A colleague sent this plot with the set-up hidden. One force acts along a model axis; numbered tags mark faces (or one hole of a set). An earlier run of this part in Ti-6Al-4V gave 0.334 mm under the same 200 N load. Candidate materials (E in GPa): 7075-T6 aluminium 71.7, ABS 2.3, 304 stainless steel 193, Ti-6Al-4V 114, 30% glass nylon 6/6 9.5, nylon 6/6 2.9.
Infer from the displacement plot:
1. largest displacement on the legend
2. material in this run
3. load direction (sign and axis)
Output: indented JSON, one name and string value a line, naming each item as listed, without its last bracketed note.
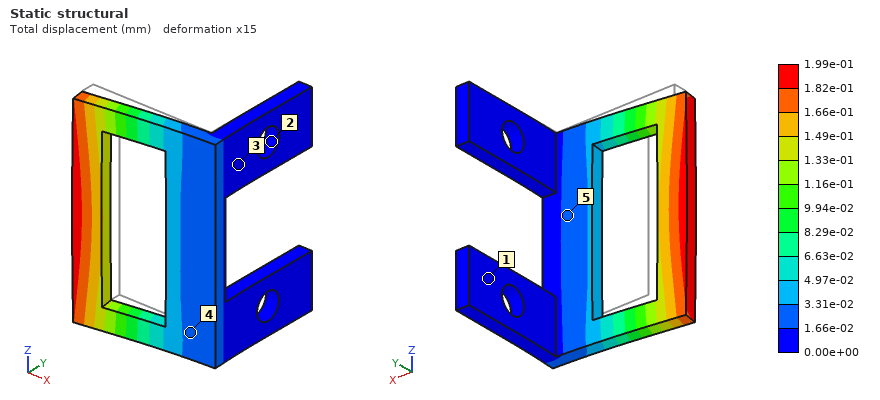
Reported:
{
  "largest displacement on the legend": "1.99e-01 mm",
  "material in this run": "304 stainless steel",
  "load direction": "-Y"
}
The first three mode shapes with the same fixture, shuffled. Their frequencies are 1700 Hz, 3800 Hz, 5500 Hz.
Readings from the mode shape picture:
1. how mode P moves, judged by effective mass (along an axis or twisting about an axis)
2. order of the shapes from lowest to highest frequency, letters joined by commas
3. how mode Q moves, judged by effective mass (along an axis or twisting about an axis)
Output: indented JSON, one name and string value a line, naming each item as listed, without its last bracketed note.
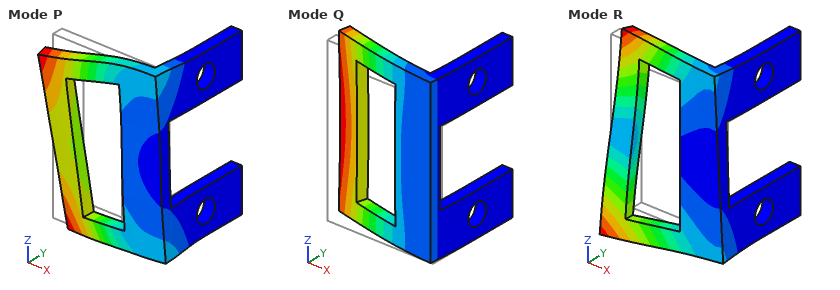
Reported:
{
  "how mode P moves, judged by effective mass": "along Z",
  "order of the shapes from lowest to highest frequency, letters joined by commas": "Q, R, P",
  "how mode Q moves, judged by effective mass": "along Y"
}
